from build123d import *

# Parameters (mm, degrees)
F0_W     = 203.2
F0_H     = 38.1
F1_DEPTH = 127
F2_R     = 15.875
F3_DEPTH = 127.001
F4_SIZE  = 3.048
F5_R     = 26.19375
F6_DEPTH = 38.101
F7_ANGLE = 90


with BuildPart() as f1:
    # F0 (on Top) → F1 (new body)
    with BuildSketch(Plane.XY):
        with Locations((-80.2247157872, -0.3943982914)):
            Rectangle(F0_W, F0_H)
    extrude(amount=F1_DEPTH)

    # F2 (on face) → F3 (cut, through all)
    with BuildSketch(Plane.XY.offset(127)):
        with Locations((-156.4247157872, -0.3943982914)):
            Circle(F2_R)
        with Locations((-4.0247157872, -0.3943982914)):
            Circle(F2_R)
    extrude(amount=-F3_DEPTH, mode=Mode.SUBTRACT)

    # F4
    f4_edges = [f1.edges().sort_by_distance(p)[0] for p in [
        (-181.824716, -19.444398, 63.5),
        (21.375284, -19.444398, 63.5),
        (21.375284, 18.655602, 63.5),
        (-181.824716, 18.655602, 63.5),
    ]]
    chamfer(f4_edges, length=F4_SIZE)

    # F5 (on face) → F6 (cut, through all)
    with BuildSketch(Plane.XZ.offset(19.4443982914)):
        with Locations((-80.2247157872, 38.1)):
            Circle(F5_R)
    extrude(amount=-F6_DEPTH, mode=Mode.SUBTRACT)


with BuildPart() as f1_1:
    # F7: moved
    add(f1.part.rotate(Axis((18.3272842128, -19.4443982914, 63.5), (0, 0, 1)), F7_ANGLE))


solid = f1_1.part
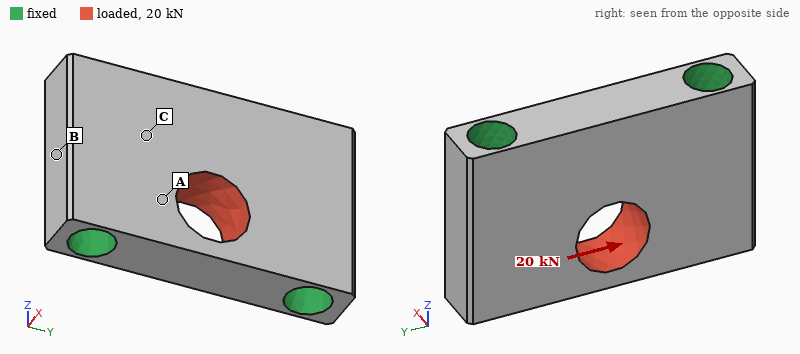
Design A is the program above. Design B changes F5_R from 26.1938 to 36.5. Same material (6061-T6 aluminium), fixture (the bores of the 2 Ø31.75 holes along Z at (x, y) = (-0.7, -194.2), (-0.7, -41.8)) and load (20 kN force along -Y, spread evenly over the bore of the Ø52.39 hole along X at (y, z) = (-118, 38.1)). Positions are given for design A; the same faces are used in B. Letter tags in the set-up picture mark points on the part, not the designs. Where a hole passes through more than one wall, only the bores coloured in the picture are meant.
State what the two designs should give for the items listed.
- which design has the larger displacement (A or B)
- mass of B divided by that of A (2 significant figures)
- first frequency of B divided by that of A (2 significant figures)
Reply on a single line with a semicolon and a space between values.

B; 0.89; 1.0
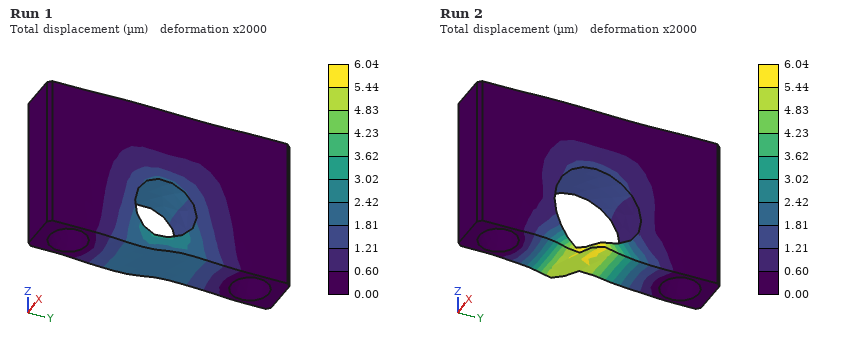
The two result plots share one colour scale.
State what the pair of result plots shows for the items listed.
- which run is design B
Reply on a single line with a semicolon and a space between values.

Run 2
